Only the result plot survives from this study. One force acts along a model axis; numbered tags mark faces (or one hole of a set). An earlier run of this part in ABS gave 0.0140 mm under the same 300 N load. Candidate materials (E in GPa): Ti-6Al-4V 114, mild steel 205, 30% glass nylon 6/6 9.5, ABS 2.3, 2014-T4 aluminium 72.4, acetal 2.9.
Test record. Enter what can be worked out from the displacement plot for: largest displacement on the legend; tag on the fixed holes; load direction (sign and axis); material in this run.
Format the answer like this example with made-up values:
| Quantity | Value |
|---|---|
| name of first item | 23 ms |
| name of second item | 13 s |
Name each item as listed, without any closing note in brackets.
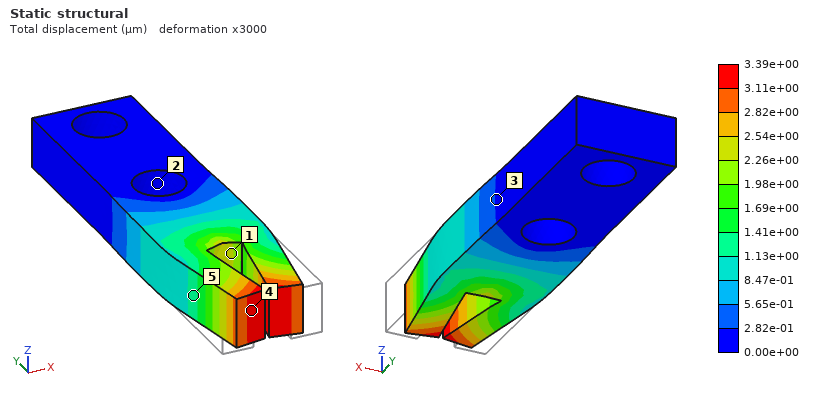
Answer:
| Quantity | Value |
|---|---|
| largest displacement on the legend | 3.39e+00 µm |
| tag on the fixed holes | 2 |
| load direction | +Y |
| material in this run | 30% glass nylon 6/6 |
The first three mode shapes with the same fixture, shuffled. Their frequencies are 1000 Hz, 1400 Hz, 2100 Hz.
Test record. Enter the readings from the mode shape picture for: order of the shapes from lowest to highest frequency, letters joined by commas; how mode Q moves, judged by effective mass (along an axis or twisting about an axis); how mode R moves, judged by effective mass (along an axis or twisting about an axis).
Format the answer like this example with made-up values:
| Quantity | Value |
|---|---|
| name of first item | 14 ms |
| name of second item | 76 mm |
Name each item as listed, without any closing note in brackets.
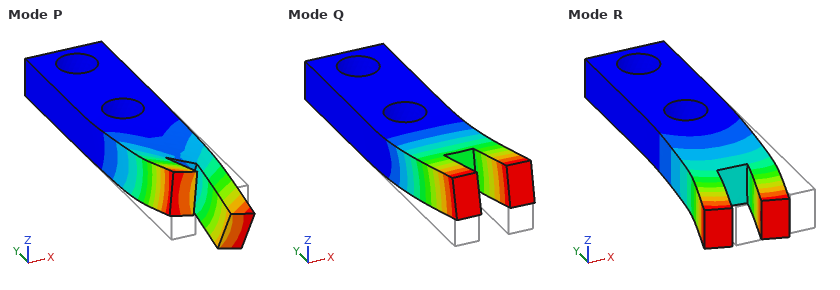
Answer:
| Quantity | Value |
|---|---|
| order of the shapes from lowest to highest frequency, letters joined by commas | Q, R, P |
| how mode Q moves, judged by effective mass | along Z |
| how mode R moves, judged by effective mass | along X |
